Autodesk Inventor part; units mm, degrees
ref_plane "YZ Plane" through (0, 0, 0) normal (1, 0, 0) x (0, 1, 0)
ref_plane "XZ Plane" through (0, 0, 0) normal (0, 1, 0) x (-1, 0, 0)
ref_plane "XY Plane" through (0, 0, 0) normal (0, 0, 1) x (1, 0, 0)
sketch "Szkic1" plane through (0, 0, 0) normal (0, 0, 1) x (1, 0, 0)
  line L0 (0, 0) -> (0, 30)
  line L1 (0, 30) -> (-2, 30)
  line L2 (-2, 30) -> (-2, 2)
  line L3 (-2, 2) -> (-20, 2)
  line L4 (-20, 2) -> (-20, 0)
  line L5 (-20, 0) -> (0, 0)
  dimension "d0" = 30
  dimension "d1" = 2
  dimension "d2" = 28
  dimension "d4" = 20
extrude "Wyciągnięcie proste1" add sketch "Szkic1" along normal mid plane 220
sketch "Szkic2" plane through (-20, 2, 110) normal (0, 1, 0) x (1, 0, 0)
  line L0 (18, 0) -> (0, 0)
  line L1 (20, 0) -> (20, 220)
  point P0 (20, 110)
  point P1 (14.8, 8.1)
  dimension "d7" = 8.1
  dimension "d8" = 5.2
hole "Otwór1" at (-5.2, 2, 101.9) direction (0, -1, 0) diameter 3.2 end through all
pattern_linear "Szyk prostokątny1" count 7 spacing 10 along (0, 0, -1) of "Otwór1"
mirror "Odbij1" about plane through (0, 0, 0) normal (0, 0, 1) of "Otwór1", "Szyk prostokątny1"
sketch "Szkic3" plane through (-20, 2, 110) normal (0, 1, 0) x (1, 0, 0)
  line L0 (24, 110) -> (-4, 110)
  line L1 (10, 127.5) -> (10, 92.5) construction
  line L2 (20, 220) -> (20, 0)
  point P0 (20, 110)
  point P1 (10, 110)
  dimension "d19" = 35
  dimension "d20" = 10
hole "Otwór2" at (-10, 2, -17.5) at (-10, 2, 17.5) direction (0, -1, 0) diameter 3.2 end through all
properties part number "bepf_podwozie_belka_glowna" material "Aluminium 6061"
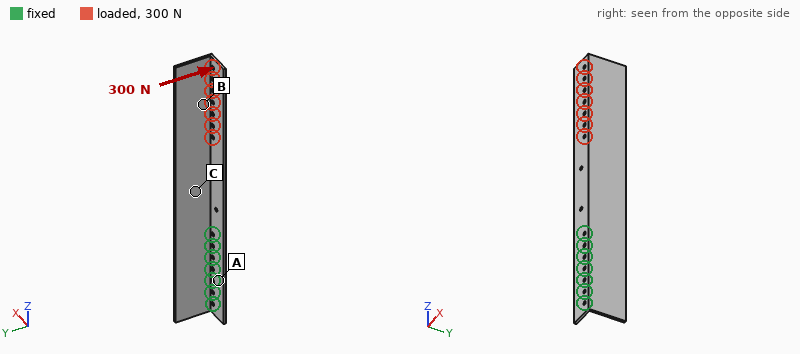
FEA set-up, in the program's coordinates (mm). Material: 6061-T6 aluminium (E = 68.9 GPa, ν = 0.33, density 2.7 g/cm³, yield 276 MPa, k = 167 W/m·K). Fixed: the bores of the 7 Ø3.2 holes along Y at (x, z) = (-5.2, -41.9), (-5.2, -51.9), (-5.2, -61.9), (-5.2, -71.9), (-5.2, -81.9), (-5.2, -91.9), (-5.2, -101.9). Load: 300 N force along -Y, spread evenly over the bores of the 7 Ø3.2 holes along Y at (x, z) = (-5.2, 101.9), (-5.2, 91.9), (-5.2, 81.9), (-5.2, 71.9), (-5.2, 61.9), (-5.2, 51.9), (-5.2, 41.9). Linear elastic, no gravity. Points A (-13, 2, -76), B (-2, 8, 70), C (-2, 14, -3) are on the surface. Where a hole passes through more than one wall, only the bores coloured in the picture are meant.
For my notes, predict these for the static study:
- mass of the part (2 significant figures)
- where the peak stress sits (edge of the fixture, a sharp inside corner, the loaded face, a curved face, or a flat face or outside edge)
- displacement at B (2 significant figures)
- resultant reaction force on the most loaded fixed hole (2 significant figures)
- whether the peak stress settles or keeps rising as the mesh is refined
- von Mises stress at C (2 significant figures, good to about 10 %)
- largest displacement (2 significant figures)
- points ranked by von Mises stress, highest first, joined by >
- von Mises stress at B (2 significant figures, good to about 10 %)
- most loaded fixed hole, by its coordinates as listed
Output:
56 g
edge of the fixture
0.64 mm
1.4 kN
keeps rising
44 MPa
1.8 mm
C > B > A
27 MPa
(-5.2, -41.9)
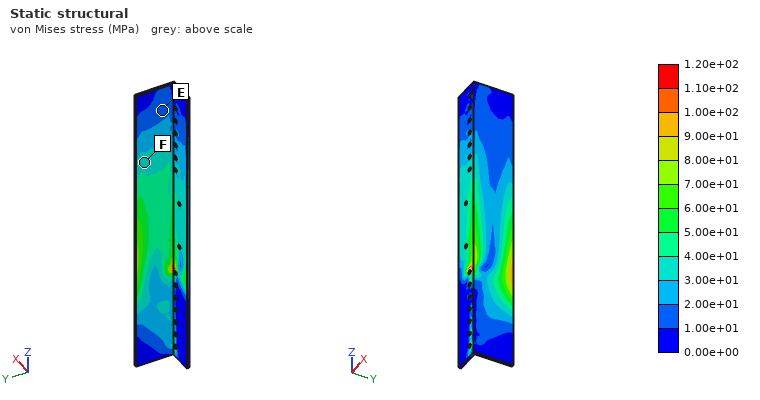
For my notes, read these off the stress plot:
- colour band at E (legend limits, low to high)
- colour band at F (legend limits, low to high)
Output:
1.00e+01 to 2.00e+01 MPa
3.00e+01 to 4.00e+01 MPa
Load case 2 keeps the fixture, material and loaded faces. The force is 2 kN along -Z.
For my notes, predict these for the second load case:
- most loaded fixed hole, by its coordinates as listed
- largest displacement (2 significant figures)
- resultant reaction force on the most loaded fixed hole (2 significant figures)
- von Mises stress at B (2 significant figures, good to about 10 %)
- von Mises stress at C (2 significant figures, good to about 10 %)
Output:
(-5.2, -41.9)
0.62 mm
1.4 kN
19 MPa
17 MPa
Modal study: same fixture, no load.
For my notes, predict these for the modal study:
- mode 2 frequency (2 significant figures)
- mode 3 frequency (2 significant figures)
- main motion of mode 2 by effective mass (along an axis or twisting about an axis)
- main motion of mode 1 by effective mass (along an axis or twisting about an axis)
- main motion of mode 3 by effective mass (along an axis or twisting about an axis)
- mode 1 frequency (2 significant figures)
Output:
560 Hz
980 Hz
along Y
along X
along Y
350 Hz
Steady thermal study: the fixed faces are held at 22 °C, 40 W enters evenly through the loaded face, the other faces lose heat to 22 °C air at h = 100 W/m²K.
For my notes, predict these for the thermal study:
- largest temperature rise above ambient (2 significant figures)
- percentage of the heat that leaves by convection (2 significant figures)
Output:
54 K
94 %
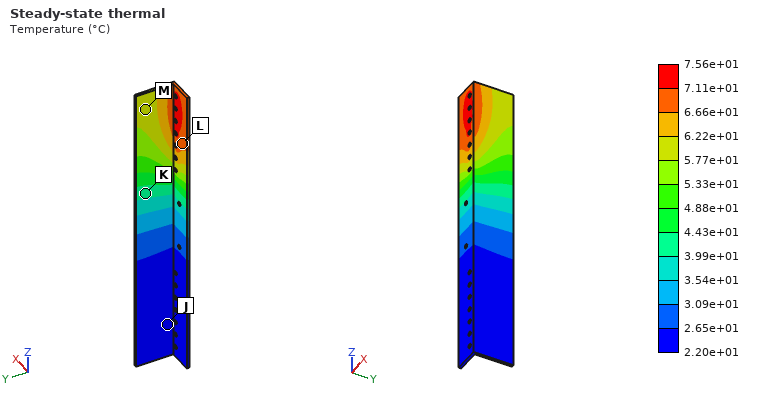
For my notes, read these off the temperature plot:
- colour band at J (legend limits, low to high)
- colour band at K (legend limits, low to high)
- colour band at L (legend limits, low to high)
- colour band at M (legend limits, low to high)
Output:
2.20e+01 to 2.65e+01 °C
3.99e+01 to 4.43e+01 °C
6.66e+01 to 7.11e+01 °C
5.77e+01 to 6.22e+01 °C
